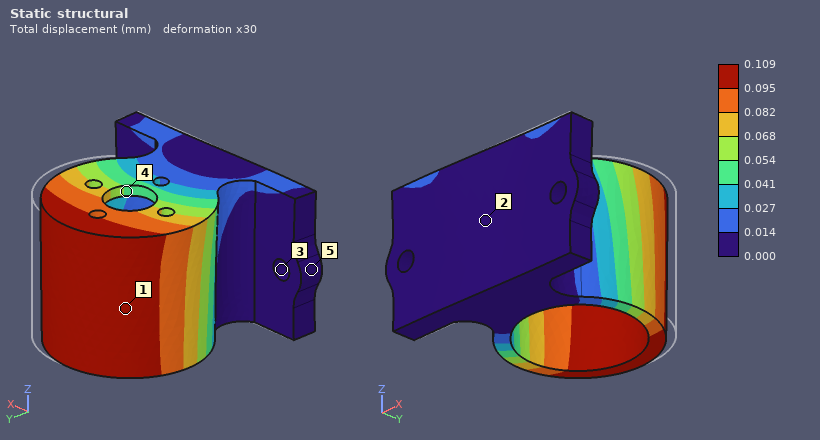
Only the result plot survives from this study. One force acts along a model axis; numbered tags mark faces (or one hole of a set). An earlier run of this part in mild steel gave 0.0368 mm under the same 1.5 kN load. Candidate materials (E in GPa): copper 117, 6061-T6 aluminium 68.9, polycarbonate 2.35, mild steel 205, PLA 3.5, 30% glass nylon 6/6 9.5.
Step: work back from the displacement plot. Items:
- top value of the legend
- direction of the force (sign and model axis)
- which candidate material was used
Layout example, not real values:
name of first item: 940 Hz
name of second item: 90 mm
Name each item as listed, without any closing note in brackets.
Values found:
top value of the legend: 0.109 mm
direction of the force: -X
which candidate material was used: 6061-T6 aluminium
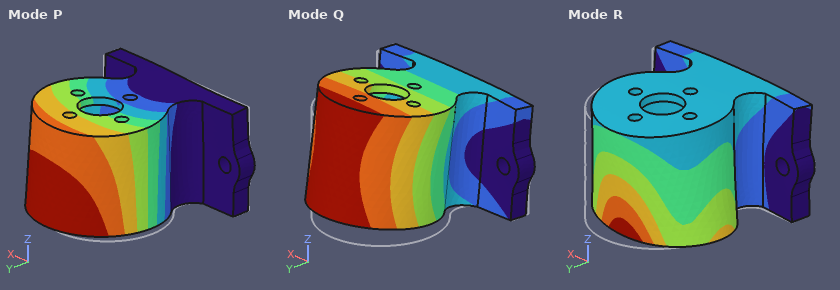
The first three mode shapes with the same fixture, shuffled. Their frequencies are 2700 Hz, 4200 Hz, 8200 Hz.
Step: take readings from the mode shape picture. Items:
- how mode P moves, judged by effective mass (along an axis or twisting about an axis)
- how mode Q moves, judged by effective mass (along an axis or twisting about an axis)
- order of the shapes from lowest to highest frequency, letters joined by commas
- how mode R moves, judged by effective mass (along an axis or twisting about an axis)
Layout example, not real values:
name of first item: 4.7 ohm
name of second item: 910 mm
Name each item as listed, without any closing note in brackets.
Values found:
how mode P moves, judged by effective mass: along X
how mode Q moves, judged by effective mass: along Z
order of the shapes from lowest to highest frequency, letters joined by commas: Q, P, R
how mode R moves, judged by effective mass: along Y
